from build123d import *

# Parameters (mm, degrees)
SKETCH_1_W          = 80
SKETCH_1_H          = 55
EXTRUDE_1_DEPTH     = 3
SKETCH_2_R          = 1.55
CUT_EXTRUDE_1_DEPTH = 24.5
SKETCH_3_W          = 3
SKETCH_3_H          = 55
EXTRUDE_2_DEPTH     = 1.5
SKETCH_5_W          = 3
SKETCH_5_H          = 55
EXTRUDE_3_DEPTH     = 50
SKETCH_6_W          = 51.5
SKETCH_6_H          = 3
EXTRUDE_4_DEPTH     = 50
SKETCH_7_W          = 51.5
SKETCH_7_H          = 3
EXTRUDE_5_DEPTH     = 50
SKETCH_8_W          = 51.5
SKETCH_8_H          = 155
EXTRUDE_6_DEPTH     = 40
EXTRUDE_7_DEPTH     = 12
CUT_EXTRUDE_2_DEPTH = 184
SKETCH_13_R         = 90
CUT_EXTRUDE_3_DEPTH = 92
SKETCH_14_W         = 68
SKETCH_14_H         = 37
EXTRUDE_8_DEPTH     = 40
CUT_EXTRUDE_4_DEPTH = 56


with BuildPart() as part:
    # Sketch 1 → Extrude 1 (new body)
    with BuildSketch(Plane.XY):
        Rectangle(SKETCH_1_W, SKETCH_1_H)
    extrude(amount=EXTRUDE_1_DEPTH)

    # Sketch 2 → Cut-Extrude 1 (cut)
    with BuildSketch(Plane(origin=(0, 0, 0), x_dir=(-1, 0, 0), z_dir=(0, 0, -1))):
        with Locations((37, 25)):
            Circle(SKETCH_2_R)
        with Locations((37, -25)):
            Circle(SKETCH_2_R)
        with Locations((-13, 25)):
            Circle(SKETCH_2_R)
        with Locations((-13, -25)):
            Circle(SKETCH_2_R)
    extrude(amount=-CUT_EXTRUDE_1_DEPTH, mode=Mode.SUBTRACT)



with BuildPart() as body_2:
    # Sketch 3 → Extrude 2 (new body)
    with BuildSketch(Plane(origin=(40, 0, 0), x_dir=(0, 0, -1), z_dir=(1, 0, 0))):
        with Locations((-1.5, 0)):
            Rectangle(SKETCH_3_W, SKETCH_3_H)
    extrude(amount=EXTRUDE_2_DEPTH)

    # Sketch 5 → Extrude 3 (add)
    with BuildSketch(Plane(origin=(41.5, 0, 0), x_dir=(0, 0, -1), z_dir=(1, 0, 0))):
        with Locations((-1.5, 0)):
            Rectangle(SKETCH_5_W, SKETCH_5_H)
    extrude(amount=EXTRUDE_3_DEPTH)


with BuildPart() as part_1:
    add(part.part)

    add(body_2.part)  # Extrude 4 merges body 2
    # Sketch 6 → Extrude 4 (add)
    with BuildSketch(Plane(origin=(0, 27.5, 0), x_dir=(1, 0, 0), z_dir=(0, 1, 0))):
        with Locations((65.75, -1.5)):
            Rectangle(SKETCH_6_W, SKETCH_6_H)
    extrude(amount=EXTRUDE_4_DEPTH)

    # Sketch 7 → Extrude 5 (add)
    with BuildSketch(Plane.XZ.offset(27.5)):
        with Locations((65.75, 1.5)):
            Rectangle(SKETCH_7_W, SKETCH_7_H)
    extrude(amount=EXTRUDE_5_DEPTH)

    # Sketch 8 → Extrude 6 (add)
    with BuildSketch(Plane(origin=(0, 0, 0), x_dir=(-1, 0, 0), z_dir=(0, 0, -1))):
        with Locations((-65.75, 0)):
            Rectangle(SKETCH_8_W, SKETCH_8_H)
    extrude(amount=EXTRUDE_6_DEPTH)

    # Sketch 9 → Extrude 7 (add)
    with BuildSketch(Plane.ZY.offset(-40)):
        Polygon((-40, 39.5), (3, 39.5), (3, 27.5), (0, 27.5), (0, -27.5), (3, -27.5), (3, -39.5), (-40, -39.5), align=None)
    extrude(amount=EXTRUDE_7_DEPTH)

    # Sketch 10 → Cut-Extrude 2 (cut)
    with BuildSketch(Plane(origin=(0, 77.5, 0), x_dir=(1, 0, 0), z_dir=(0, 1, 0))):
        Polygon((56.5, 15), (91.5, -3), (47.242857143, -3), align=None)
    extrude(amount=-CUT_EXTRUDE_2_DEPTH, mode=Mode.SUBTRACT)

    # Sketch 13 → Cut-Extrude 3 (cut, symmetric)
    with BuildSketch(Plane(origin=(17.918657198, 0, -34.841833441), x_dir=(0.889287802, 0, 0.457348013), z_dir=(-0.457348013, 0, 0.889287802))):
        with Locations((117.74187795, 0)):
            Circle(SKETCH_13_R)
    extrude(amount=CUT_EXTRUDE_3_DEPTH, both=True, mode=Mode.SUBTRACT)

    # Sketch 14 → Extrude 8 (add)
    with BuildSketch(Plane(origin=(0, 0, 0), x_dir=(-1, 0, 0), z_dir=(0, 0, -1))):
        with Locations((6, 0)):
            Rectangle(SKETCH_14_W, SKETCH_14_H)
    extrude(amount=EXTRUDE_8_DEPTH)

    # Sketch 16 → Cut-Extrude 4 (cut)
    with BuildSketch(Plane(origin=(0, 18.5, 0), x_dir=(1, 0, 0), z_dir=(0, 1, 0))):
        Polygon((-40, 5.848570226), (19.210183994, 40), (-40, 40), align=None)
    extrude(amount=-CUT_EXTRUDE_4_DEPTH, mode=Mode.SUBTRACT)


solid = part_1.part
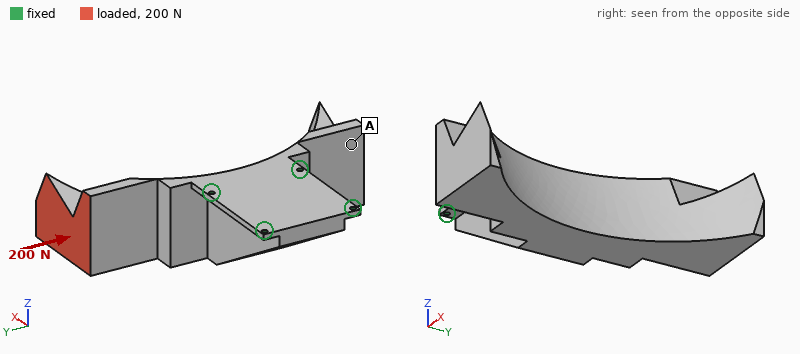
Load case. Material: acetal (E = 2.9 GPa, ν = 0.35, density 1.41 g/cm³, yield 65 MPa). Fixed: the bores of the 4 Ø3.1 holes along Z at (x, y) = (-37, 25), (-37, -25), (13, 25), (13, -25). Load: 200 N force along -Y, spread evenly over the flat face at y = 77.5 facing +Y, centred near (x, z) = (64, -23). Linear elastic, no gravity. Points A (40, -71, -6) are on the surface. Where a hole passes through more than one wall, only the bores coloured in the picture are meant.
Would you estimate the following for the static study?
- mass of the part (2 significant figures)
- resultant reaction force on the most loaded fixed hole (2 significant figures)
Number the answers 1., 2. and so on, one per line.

1. 290 g
2. 200 N
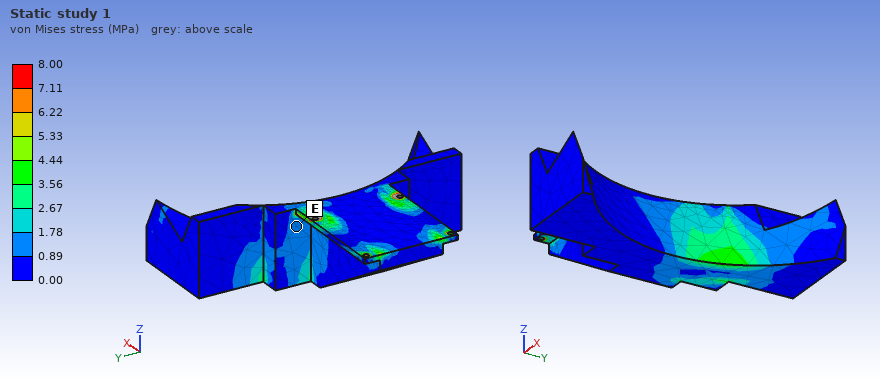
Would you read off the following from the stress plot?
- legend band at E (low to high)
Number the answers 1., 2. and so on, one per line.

1. 0.89 to 1.78 MPa
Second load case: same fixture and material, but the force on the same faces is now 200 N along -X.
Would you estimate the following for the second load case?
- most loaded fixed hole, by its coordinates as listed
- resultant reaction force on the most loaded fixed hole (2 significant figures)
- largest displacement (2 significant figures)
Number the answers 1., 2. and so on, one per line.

1. (13, 25)
2. 240 N
3. 1.0 mm
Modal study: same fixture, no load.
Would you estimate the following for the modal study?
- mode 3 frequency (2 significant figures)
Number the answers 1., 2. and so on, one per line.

1. 380 Hz
